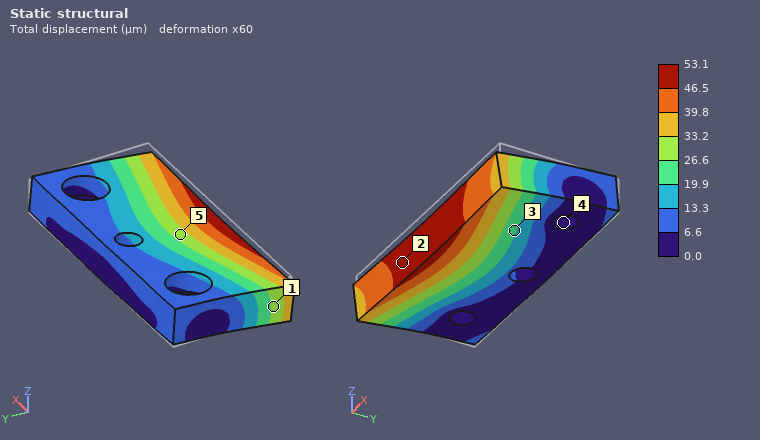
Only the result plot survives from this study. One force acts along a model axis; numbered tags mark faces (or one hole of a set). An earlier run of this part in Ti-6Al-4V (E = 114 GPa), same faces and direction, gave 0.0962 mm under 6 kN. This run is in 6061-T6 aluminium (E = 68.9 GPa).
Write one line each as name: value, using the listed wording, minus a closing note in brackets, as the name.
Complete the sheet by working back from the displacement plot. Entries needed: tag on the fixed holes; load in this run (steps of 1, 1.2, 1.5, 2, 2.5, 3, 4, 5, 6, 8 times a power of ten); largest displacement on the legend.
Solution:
tag on the fixed holes: 4
load in this run: 2 kN
largest displacement on the legend: 53.1 µm
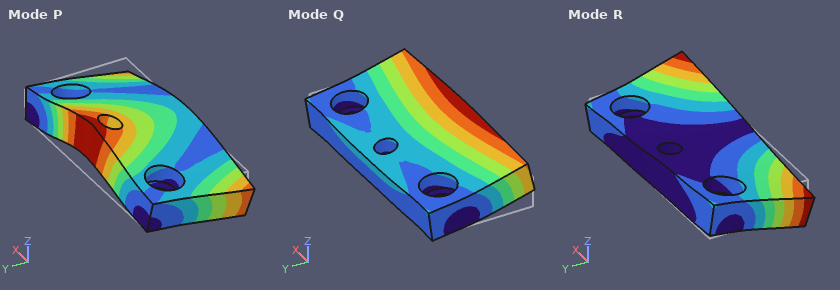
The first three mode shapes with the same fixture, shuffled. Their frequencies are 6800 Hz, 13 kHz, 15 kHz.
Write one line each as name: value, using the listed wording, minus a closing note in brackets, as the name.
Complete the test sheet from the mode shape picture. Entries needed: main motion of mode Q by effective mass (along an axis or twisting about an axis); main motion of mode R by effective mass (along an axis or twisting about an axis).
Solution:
main motion of mode Q by effective mass: along Z
main motion of mode R by effective mass: twisting about Y
